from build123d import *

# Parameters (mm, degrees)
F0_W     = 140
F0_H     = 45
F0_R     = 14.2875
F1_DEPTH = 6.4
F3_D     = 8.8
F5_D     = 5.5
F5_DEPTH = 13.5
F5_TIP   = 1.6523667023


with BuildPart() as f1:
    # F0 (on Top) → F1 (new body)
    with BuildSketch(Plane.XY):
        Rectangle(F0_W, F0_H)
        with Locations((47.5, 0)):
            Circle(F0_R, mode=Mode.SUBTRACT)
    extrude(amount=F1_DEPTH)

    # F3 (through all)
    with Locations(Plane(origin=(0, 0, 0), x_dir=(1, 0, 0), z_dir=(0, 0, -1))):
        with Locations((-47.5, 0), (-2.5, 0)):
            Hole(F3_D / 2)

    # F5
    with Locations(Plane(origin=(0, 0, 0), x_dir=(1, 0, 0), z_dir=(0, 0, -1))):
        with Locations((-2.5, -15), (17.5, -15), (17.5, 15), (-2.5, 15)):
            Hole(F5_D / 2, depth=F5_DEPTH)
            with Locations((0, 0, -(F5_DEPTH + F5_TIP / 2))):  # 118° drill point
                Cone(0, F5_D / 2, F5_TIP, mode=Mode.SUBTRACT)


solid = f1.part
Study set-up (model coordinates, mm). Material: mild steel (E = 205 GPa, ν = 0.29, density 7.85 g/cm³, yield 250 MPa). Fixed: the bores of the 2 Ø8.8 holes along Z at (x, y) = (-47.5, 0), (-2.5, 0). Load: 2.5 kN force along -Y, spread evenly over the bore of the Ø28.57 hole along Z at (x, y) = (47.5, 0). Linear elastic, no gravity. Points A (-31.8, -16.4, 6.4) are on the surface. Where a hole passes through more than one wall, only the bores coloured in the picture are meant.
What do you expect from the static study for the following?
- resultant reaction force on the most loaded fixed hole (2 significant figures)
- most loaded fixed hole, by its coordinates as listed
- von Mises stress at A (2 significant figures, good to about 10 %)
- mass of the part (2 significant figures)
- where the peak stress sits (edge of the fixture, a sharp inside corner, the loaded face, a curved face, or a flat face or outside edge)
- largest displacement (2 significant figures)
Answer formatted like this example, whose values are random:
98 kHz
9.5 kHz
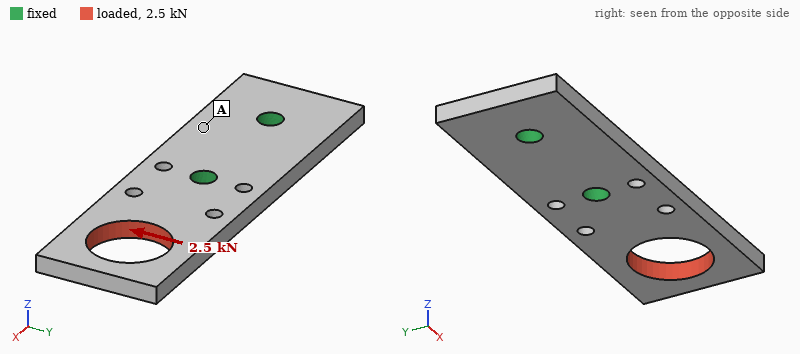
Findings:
4.4 kN
(-2.5, 0)
15 MPa
270 g
edge of the fixture
67 µm
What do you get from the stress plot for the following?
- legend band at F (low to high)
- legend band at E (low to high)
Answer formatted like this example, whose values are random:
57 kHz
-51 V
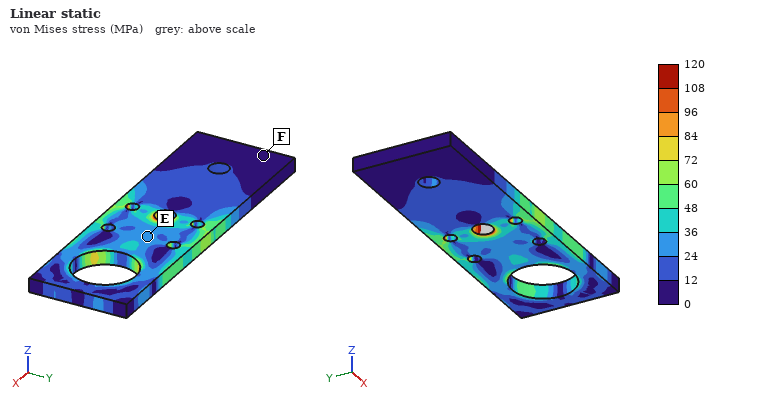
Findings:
0 to 12 MPa
24 to 36 MPa
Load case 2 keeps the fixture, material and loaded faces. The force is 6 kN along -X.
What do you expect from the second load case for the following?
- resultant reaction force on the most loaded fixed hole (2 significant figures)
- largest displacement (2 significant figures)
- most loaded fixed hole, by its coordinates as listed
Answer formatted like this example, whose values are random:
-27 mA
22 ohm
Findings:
5.0 kN
17 µm
(-2.5, 0)
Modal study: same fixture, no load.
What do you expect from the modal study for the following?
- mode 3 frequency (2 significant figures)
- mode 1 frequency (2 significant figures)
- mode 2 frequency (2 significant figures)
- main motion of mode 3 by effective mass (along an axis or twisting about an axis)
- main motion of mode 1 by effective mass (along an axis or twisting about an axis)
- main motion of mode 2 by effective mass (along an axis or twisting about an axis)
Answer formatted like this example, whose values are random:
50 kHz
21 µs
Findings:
4100 Hz
1100 Hz
2800 Hz
along Y
along Z
twisting about X
